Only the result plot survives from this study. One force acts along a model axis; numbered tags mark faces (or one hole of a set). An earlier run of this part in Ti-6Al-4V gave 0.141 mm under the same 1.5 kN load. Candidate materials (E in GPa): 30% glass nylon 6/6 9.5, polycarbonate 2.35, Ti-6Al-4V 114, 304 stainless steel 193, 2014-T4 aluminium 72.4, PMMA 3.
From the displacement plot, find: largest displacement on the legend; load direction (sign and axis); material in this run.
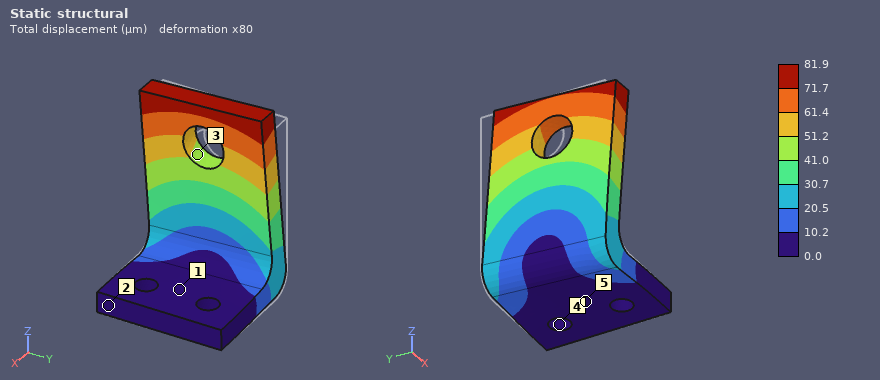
81.9 µm
-Y
304 stainless steel
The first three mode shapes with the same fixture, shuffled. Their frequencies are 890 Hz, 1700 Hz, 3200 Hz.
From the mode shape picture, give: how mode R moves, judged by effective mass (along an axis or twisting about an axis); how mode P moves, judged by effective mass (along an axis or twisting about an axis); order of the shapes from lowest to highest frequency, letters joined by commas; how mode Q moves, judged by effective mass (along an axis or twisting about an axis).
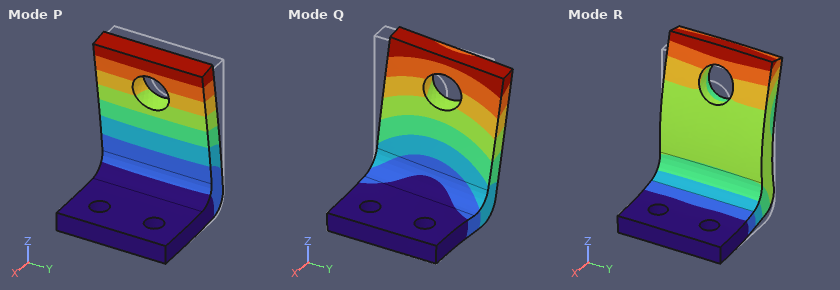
along Z
along X
P, Q, R
along Y
